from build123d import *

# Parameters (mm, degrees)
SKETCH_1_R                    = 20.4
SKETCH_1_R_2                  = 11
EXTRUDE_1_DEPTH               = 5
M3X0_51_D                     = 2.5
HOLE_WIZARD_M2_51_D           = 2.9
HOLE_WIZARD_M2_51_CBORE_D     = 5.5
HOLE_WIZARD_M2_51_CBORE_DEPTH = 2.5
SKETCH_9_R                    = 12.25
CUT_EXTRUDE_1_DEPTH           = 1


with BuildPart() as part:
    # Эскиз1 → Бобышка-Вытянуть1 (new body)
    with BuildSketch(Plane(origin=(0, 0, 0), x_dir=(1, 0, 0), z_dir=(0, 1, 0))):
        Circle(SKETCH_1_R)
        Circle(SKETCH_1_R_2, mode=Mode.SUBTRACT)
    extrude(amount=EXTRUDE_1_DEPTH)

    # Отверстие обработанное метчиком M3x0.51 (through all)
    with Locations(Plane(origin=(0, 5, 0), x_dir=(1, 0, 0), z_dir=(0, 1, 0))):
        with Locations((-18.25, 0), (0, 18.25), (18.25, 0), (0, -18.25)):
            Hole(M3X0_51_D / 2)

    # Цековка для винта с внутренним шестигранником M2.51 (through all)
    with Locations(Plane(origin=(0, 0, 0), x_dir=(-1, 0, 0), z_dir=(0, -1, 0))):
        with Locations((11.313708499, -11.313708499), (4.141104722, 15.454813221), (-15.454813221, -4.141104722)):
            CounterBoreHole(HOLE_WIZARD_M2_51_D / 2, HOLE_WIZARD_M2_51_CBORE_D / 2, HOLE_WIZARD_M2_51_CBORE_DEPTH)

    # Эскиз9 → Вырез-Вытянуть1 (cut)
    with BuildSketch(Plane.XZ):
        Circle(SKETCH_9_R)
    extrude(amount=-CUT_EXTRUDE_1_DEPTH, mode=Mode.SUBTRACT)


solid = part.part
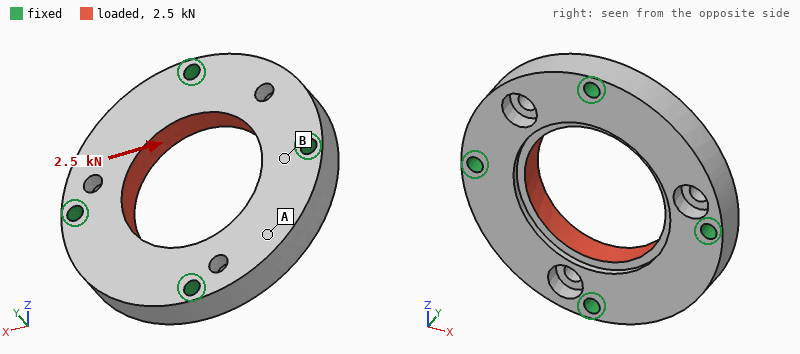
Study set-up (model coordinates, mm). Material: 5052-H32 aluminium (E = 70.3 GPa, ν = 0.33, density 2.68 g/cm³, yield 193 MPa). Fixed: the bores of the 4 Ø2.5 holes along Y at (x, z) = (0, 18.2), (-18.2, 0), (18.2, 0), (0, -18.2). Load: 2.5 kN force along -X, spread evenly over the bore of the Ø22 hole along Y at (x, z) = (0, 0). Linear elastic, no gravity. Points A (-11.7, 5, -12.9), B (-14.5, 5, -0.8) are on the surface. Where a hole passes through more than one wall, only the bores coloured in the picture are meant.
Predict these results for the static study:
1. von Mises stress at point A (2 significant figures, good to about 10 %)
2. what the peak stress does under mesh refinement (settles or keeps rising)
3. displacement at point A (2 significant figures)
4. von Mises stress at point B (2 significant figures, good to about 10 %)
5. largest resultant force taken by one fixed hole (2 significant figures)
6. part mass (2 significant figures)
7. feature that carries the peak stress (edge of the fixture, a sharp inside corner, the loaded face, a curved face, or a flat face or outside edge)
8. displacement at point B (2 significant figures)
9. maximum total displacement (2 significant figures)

7.5 MPa
keeps rising
3.5 µm
22 MPa
690 N
11 g
edge of the fixture
1.0 µm
4.3 µm
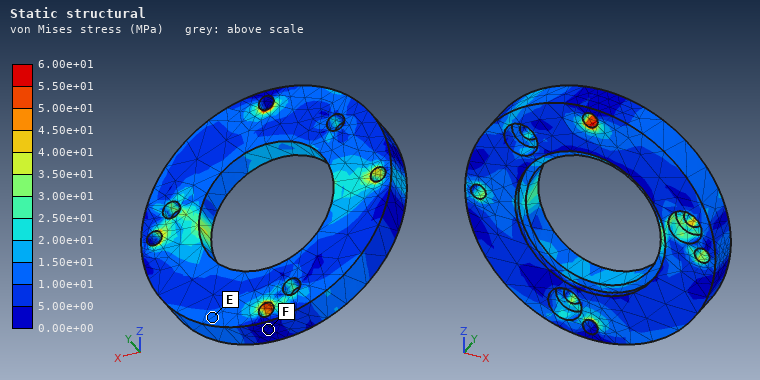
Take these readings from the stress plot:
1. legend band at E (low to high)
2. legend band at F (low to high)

1.00e+01 to 1.50e+01 MPa
0.00e+00 to 5.00e+00 MPa
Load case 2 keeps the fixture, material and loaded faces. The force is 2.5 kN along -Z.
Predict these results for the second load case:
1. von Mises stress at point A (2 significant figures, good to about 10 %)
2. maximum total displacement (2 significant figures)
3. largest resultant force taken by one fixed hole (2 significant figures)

7.8 MPa
4.4 µm
690 N
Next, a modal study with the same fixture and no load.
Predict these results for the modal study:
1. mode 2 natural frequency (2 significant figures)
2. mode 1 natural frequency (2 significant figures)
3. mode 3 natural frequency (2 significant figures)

26 kHz
25 kHz
28 kHz
